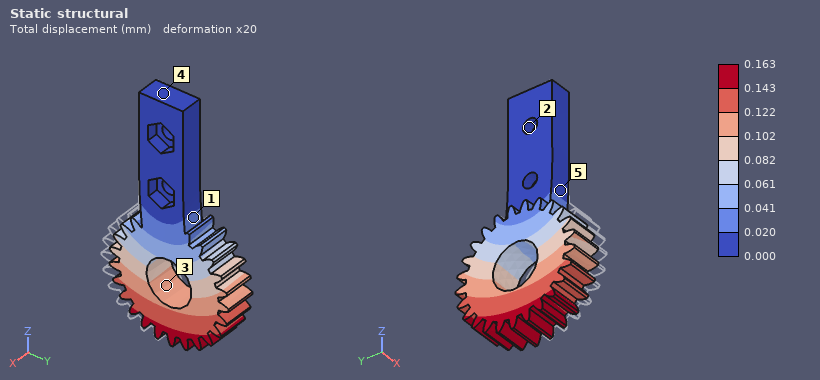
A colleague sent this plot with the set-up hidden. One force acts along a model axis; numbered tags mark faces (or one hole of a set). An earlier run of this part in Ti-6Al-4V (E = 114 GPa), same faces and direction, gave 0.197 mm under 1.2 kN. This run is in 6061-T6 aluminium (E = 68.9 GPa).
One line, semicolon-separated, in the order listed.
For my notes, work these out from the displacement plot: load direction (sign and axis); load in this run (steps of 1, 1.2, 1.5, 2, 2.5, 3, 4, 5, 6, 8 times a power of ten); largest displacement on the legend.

+Y; 600 N; 0.163 mm
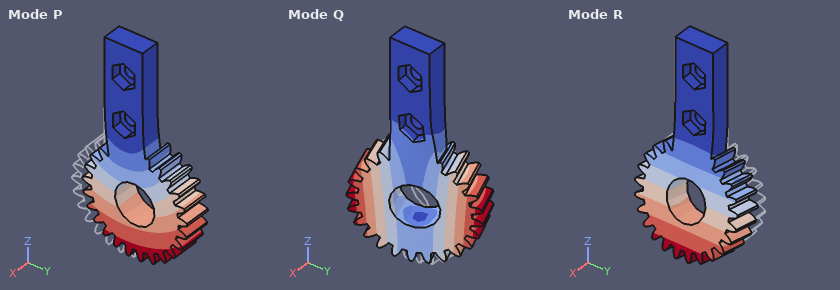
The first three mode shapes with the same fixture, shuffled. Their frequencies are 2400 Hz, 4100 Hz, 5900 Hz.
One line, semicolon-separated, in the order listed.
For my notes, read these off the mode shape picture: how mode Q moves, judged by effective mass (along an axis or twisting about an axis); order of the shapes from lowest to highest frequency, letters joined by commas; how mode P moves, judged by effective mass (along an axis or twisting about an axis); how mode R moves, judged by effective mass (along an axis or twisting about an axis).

twisting about Z; R, P, Q; along Y; along X
